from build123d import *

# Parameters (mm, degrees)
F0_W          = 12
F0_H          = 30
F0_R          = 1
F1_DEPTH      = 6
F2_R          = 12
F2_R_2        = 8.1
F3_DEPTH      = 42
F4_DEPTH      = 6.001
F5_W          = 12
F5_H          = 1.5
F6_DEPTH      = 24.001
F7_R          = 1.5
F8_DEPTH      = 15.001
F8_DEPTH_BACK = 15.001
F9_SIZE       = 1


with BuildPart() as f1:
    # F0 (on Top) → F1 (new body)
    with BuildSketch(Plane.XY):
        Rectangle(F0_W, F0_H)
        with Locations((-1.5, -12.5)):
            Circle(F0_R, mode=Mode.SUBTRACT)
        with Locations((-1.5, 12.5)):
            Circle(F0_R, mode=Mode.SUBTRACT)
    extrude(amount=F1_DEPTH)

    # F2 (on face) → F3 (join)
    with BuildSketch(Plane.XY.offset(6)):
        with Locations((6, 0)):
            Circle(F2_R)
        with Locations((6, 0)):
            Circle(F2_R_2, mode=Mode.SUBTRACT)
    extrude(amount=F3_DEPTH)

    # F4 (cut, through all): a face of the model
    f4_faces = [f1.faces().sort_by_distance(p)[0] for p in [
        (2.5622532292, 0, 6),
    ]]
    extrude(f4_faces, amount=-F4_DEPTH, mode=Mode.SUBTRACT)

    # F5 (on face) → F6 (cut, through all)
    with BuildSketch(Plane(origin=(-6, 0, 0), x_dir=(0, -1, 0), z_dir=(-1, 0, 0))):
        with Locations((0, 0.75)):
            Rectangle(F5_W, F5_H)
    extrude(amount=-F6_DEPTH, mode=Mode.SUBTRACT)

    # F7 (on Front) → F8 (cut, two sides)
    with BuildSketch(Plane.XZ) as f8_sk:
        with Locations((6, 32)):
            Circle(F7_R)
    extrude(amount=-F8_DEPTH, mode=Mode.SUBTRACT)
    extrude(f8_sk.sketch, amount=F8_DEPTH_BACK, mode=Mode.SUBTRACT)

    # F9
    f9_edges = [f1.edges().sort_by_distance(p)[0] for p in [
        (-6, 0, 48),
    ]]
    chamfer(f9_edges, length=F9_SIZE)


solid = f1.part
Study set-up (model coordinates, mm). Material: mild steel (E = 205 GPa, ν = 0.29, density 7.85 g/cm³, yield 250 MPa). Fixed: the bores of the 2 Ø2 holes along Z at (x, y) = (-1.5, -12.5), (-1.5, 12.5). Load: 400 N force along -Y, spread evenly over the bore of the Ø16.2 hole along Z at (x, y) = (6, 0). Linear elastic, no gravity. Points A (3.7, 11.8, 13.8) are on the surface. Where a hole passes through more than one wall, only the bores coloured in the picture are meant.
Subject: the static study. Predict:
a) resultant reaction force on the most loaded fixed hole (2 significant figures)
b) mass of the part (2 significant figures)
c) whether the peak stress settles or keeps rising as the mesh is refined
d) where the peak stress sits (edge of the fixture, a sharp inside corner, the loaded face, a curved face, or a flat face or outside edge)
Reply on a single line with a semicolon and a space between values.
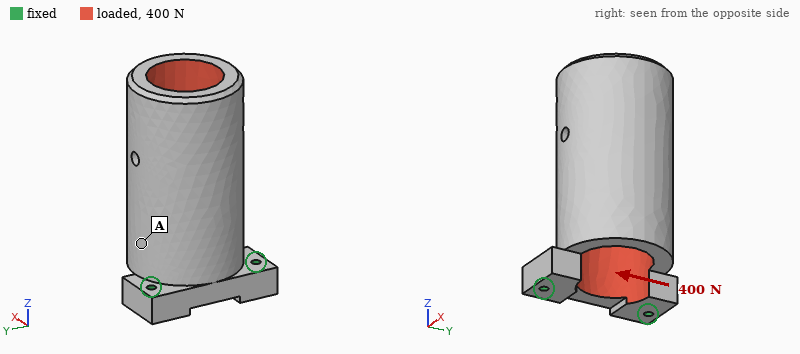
460 N; 92 g; keeps rising; edge of the fixture
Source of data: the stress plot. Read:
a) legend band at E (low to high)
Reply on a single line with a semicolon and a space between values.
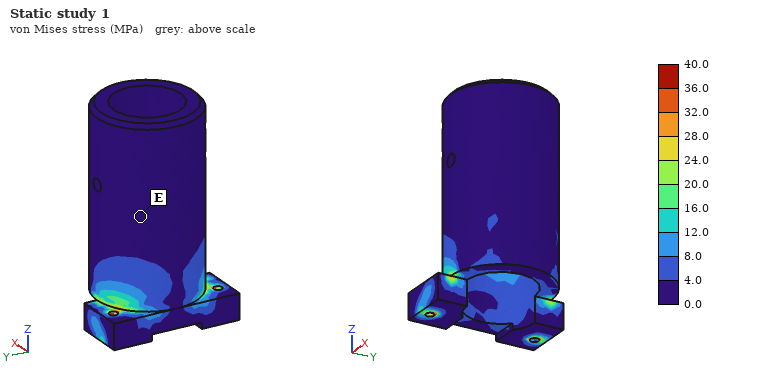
0.0 to 4.0 MPa
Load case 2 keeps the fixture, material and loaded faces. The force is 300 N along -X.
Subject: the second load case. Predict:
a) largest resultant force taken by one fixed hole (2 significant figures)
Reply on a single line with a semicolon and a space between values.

150 N
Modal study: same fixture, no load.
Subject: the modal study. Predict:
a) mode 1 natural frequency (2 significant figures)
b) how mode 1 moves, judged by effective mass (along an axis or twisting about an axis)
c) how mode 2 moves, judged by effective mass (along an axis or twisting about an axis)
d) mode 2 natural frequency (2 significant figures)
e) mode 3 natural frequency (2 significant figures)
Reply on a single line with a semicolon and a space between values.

1900 Hz; along X; along Y; 5200 Hz; 9300 Hz
